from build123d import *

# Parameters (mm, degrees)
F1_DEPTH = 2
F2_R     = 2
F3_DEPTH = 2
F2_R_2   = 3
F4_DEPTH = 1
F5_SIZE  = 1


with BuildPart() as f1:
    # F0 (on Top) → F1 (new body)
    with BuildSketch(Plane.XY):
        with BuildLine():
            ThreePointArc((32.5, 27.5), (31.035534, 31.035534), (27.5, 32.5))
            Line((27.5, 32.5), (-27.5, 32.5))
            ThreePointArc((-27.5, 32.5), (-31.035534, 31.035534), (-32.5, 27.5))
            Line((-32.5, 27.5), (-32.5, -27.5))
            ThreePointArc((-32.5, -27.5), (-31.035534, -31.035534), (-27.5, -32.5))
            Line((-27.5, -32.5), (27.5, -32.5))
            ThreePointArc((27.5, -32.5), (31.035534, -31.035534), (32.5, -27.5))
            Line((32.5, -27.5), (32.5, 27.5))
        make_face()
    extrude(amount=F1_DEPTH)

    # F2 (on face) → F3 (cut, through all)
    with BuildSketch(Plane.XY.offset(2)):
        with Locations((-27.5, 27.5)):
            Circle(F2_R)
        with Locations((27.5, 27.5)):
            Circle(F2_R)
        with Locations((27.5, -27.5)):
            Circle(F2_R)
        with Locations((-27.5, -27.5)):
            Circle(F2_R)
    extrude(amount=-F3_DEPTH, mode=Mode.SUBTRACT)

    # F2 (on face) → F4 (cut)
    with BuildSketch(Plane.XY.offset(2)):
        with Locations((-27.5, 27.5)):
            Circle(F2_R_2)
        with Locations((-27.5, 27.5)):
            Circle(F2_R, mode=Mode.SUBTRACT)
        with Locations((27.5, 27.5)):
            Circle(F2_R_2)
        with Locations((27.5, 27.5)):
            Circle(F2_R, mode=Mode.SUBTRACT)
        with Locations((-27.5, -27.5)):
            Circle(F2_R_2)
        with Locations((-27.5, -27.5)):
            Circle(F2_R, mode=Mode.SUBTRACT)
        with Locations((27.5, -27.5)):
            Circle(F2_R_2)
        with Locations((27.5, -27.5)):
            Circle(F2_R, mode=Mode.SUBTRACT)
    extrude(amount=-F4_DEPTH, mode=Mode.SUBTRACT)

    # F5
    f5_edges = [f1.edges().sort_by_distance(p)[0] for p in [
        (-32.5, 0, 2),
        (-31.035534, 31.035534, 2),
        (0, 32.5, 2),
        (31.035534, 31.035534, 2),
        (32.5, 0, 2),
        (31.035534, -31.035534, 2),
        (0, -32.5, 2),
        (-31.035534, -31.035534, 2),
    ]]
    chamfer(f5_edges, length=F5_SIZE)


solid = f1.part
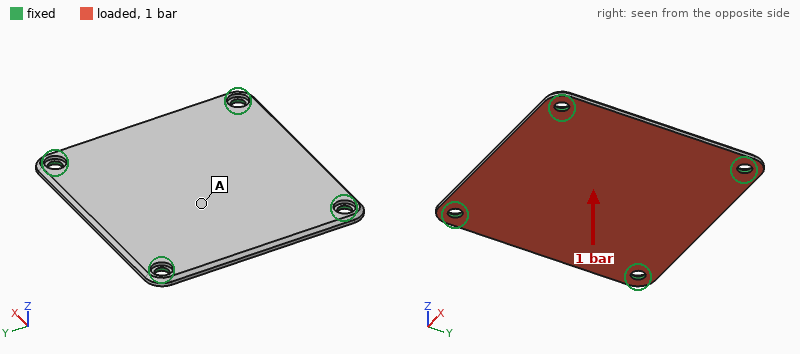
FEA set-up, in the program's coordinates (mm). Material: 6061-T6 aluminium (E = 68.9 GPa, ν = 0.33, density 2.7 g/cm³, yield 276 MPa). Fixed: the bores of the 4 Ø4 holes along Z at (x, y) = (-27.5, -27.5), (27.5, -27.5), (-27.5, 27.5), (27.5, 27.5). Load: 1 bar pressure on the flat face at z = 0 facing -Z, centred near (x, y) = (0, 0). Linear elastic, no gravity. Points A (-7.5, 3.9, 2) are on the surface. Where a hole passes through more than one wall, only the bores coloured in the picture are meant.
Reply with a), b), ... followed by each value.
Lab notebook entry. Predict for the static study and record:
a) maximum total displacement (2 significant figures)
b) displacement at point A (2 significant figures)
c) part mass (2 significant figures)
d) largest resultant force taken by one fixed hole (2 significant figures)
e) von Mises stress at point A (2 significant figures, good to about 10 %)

a) 0.16 mm
b) 0.15 mm
c) 22 g
d) 220 N
e) 27 MPa
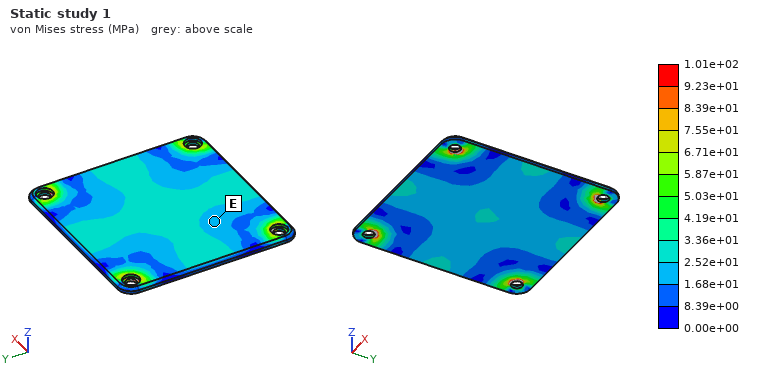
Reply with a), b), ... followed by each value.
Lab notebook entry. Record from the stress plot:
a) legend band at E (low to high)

a) 1.68e+01 to 2.52e+01 MPa
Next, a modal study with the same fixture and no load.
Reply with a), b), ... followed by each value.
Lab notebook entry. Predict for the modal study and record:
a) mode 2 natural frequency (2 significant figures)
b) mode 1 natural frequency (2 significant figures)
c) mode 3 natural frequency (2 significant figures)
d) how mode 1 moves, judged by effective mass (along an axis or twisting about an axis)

a) 3500 Hz
b) 2100 Hz
c) 3500 Hz
d) along Z
